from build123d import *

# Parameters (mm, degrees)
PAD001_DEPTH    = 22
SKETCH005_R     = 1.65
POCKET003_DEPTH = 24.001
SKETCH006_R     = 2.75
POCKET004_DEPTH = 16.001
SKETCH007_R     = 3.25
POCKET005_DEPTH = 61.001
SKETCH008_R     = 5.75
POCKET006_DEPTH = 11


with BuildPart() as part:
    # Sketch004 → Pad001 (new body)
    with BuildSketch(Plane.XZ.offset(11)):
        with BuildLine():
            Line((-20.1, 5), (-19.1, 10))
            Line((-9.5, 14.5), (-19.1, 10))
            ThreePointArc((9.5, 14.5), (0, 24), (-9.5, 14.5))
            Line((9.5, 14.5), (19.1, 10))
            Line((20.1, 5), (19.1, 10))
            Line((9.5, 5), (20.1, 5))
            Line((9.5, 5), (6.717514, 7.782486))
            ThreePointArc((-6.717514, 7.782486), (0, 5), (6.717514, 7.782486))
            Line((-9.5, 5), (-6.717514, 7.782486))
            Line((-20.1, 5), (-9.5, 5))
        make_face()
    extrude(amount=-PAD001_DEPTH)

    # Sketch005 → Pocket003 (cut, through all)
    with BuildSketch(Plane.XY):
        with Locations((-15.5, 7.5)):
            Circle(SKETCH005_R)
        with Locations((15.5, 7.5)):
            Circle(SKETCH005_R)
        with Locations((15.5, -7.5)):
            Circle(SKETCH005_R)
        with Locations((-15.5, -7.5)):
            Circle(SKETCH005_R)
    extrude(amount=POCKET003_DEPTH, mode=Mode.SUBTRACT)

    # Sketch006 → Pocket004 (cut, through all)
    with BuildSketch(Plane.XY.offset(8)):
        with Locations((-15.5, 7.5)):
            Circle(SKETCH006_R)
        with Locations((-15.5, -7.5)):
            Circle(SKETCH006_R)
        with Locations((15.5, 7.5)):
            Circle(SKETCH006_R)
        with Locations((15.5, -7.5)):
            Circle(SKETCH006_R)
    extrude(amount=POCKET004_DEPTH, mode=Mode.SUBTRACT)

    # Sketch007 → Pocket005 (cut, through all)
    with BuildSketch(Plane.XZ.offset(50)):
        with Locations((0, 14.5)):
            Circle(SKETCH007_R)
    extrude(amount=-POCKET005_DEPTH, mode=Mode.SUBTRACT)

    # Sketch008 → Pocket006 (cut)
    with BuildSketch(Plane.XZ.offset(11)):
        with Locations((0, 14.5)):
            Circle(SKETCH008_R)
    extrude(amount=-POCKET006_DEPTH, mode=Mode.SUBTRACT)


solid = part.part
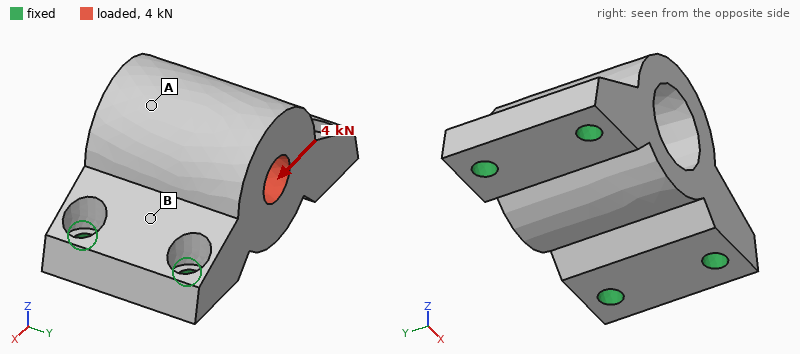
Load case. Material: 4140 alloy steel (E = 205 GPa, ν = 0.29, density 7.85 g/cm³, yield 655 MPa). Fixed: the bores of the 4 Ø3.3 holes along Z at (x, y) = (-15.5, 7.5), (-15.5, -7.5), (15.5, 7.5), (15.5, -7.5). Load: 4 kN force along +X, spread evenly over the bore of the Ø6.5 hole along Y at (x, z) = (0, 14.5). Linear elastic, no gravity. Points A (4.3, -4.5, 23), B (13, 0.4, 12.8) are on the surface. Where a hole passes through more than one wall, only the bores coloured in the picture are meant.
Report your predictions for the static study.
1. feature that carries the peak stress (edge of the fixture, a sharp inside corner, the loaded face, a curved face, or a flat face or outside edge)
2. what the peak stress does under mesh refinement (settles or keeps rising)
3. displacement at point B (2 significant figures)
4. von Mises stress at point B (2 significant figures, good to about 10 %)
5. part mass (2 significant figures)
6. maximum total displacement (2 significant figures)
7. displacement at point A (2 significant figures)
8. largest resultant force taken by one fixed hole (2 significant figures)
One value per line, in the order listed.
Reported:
edge of the fixture
keeps rising
1.7 µm
15 MPa
62 g
4.0 µm
2.3 µm
1.4 kN
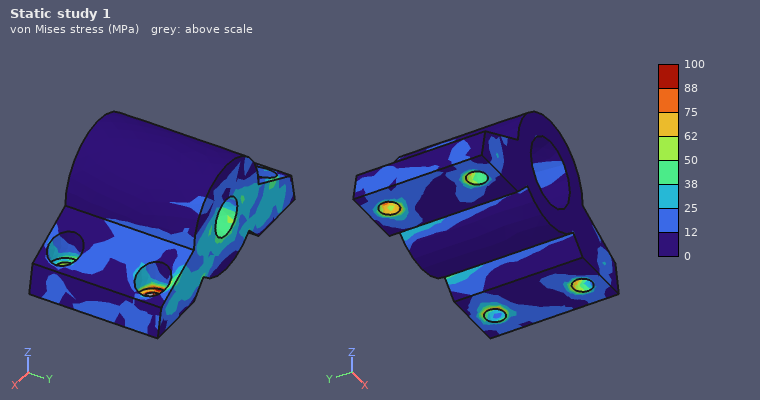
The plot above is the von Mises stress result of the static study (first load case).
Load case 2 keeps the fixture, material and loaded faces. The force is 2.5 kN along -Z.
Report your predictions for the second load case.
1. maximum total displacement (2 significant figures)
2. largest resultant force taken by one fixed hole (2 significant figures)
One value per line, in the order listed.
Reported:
5.3 µm
1.3 kN
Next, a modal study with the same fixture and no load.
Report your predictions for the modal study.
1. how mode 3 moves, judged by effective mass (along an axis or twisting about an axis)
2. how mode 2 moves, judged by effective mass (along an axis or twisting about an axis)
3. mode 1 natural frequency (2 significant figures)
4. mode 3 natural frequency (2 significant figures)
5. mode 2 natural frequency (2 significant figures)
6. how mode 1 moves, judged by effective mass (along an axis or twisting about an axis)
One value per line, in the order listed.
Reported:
along X
along Z
19 kHz
29 kHz
24 kHz
along Y
